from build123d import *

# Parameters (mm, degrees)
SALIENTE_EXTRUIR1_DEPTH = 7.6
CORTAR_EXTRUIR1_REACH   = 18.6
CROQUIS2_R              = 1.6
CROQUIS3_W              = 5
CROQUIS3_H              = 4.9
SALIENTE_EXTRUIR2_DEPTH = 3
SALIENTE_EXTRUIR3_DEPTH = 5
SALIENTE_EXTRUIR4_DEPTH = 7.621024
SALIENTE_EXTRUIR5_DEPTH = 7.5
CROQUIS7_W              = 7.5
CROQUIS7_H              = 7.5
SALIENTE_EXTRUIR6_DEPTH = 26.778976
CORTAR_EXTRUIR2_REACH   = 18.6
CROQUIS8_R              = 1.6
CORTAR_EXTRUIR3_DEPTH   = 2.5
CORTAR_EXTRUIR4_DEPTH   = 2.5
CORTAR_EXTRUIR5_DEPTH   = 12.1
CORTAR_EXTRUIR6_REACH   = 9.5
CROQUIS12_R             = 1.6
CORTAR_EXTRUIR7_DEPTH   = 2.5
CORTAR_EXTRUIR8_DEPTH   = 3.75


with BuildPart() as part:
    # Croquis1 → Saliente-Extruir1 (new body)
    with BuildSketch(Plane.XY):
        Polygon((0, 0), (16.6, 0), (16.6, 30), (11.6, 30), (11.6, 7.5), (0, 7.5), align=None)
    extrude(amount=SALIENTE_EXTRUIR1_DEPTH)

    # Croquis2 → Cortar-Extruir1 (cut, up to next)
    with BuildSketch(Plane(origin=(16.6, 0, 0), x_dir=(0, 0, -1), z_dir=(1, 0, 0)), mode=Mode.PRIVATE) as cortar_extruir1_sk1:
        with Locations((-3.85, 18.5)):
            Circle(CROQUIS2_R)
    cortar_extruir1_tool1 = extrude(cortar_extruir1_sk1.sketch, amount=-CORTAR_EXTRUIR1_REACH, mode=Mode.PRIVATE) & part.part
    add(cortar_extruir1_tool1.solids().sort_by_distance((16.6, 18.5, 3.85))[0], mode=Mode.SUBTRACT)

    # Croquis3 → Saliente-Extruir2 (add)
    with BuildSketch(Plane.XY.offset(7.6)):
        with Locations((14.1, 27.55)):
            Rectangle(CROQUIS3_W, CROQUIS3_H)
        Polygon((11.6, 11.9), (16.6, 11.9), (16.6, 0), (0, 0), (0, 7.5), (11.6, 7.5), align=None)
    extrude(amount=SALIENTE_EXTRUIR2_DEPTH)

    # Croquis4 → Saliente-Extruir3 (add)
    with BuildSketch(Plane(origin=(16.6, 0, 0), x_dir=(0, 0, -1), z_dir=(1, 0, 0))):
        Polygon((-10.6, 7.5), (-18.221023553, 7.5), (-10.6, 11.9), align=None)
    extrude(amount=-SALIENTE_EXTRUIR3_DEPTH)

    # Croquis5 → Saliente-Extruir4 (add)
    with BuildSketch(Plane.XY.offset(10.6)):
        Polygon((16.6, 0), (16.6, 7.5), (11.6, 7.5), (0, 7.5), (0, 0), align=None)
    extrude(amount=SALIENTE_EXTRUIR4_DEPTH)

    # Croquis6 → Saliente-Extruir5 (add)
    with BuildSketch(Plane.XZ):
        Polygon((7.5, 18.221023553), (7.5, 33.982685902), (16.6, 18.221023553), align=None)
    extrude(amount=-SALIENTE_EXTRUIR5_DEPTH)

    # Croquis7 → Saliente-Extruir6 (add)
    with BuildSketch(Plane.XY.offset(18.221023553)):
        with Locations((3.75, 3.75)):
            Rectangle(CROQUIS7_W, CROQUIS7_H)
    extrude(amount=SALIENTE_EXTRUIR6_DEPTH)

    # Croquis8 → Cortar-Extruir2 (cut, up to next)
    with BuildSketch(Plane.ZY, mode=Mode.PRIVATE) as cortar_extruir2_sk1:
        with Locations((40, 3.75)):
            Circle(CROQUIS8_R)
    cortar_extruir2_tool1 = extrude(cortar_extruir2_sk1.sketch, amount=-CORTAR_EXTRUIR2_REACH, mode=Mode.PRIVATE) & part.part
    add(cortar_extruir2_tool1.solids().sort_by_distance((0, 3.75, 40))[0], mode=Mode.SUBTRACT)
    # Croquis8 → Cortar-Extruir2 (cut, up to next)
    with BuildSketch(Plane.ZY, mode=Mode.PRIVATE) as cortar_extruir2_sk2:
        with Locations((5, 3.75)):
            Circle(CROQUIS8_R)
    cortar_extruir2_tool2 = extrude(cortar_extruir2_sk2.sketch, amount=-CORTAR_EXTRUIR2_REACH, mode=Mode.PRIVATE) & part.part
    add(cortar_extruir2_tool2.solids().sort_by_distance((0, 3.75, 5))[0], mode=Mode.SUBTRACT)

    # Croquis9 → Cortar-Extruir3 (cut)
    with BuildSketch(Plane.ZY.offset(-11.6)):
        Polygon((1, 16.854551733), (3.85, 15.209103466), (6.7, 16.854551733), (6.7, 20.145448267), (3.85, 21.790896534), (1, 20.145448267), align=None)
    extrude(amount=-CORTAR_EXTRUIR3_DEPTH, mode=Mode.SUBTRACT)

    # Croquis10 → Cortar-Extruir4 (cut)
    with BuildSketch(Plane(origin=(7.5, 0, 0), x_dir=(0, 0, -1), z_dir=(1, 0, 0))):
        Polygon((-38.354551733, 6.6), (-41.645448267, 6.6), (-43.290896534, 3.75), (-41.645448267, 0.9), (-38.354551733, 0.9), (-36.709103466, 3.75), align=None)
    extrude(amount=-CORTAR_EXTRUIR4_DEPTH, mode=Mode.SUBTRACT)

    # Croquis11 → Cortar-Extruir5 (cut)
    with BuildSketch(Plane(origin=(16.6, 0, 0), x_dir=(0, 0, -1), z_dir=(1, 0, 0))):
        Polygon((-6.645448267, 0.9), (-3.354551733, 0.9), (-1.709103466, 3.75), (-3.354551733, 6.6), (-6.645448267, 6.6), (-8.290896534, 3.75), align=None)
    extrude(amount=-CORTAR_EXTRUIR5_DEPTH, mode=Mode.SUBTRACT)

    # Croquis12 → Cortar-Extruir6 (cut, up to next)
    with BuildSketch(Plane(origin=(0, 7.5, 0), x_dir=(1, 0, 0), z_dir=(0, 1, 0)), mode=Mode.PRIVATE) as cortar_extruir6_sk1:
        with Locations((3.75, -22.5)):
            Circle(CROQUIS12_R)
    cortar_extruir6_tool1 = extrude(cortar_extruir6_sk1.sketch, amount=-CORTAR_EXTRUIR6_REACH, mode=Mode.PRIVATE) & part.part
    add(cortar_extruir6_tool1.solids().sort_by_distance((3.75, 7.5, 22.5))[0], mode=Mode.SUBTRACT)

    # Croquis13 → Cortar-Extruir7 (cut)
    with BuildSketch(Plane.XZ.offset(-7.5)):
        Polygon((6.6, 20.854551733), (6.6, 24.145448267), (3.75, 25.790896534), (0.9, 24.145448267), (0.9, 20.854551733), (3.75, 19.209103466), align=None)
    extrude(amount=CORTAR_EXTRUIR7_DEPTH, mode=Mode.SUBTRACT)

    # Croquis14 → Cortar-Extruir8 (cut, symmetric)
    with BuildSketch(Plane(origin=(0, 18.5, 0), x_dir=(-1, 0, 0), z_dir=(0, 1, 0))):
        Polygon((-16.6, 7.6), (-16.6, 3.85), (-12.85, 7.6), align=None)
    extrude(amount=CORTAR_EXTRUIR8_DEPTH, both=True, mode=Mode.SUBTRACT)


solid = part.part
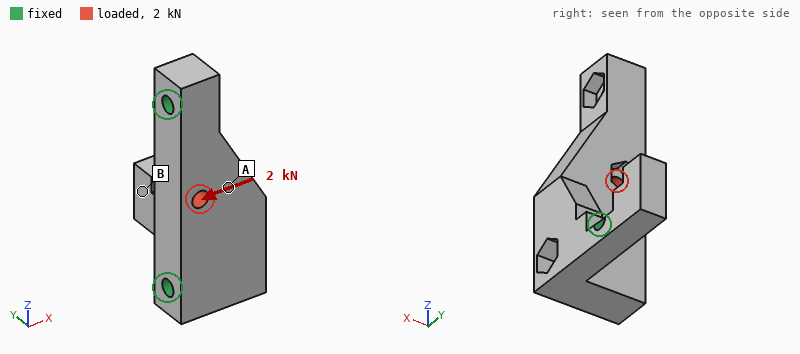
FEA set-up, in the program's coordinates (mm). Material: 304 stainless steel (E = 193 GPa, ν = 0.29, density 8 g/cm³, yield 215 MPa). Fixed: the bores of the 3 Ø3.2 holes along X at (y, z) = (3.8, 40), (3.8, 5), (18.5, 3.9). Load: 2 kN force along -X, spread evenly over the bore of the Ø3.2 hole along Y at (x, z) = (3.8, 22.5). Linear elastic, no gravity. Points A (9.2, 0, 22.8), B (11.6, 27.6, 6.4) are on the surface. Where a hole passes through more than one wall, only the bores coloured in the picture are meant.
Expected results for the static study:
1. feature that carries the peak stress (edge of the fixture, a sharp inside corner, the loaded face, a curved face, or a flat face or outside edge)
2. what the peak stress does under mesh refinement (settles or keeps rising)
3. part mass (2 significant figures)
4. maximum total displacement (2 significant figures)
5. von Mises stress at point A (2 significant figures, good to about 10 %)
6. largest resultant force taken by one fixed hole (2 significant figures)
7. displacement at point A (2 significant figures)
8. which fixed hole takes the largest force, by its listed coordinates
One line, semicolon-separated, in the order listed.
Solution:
edge of the fixture; keeps rising; 37 g; 8.9 µm; 45 MPa; 1.3 kN; 6.9 µm; (3.8, 5)
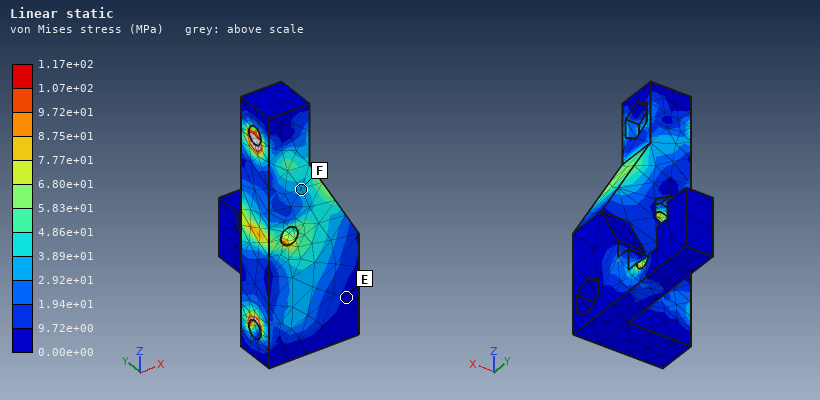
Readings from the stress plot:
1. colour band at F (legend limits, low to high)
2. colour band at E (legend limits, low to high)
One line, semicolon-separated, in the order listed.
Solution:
2.92e+01 to 3.89e+01 MPa; 0.00e+00 to 9.72e+00 MPa
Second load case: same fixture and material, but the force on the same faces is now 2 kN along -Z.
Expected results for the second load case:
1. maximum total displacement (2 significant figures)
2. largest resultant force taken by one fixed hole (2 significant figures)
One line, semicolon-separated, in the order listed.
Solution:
2.3 µm; 980 N
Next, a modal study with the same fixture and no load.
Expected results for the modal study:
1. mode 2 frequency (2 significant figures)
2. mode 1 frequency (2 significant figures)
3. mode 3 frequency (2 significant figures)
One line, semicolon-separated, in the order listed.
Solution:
18 kHz; 13 kHz; 18 kHz
